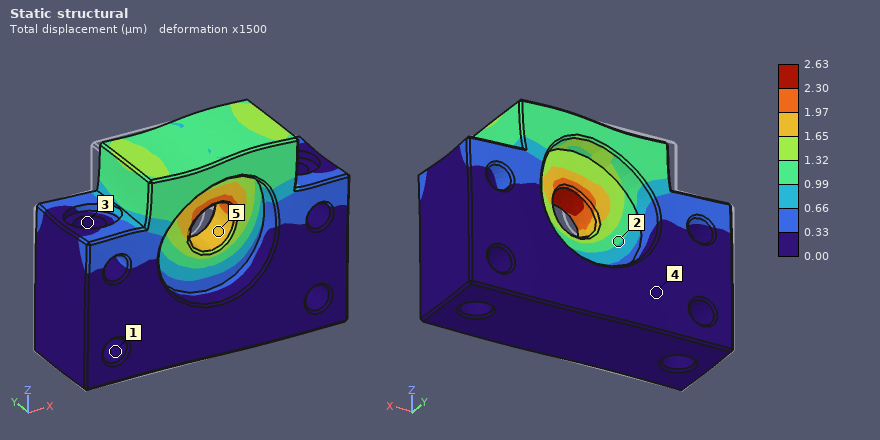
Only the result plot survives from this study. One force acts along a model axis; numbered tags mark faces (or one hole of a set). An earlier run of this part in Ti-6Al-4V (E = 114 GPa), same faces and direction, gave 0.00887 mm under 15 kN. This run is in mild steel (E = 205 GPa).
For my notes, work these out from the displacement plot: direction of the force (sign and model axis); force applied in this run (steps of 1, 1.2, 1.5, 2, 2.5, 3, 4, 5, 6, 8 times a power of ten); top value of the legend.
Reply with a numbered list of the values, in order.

1. +X
2. 8 kN
3. 2.63 µm
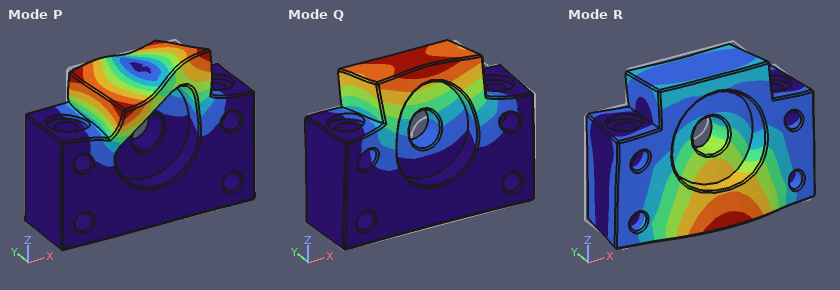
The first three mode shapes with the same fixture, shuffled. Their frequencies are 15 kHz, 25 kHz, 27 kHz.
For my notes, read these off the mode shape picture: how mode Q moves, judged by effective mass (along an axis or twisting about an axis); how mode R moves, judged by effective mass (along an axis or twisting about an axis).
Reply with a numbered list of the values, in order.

1. along Y
2. along Y
